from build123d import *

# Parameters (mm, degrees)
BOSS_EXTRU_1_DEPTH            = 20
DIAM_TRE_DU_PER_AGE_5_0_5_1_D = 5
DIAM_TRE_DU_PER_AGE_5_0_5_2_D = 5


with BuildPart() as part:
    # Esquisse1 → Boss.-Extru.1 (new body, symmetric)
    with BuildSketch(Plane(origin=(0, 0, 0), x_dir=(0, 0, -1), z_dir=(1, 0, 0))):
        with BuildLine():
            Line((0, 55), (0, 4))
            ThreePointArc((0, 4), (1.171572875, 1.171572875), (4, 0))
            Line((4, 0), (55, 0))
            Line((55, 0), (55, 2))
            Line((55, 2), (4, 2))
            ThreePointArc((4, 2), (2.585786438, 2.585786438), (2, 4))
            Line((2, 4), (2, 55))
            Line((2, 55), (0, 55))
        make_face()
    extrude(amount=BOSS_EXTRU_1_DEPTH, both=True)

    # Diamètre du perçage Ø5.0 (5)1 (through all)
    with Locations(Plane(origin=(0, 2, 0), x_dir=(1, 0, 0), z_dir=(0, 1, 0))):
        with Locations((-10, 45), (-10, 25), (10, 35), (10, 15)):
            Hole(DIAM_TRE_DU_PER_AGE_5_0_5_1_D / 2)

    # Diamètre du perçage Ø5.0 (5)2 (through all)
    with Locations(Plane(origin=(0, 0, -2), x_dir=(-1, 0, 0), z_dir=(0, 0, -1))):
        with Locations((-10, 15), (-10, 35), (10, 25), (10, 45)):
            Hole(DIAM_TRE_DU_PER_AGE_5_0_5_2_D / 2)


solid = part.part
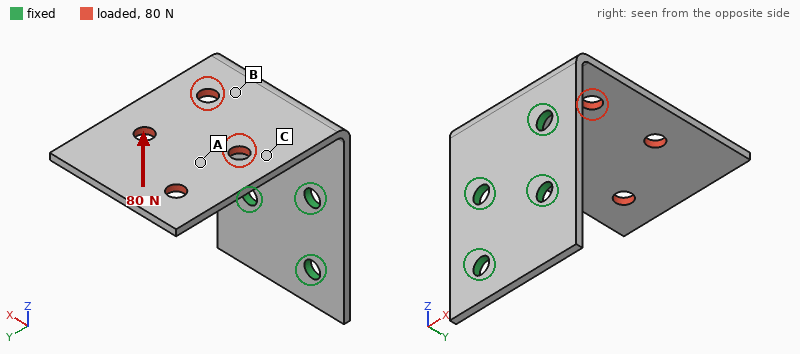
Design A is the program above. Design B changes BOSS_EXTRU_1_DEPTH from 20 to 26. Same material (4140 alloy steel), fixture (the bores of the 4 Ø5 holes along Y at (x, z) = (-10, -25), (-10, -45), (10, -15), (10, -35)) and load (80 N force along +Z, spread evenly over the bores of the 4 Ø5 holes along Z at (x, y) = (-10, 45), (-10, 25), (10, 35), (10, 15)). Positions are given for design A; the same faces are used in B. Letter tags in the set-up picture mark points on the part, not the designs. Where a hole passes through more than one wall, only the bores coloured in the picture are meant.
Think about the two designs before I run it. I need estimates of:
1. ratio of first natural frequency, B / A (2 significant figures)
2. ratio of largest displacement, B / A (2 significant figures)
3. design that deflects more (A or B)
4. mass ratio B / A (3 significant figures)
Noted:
0.99
0.78
A
1.31
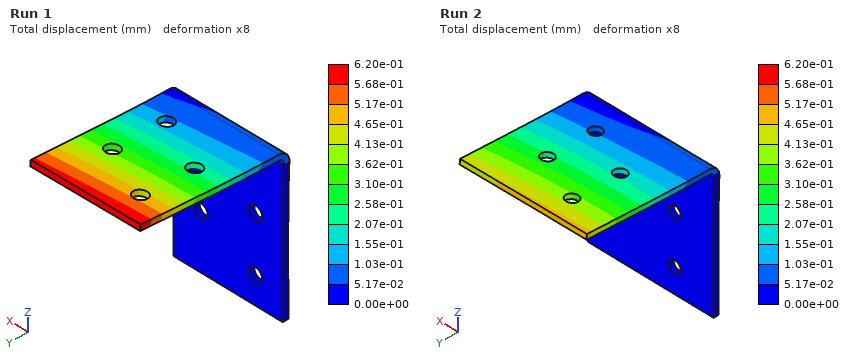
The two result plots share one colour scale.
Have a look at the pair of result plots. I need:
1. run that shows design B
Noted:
Run 2
